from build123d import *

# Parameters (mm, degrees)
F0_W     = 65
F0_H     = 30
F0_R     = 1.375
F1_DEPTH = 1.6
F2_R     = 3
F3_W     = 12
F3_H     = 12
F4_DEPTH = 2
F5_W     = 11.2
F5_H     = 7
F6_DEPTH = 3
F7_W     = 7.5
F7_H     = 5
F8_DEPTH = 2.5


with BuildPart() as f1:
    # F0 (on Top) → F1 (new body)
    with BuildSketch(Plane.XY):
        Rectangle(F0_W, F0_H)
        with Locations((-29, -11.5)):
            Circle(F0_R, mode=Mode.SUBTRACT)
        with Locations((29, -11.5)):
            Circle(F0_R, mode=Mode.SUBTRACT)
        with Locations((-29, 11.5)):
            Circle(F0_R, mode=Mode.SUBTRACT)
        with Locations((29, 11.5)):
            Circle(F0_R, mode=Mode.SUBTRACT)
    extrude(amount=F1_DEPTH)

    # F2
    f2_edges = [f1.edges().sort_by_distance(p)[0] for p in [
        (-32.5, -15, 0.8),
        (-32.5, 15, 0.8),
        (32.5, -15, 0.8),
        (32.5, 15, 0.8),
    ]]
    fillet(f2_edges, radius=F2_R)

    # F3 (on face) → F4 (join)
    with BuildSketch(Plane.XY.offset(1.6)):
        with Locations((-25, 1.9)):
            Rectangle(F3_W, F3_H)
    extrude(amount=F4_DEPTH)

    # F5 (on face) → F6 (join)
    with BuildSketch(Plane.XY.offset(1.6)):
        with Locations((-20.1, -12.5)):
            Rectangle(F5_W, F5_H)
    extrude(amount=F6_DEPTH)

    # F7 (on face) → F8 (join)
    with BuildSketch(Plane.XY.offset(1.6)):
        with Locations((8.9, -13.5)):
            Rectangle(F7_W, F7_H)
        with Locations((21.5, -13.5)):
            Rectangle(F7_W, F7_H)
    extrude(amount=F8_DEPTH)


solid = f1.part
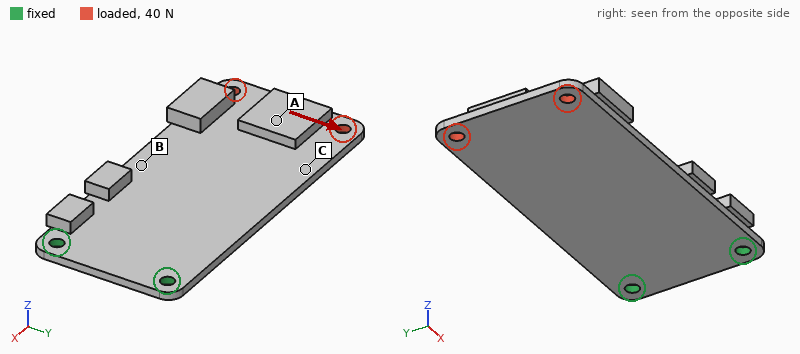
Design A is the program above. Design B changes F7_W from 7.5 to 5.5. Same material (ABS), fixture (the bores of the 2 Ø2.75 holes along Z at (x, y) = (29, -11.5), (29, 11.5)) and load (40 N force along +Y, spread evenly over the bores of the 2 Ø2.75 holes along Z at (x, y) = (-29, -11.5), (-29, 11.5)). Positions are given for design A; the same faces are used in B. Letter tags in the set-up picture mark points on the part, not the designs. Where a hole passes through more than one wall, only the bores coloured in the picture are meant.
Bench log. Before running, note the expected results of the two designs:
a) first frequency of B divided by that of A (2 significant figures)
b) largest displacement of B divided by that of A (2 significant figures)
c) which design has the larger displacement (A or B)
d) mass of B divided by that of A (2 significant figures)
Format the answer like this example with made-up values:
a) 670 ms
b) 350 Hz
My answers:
a) 0.97
b) 0.92
c) A
d) 0.99
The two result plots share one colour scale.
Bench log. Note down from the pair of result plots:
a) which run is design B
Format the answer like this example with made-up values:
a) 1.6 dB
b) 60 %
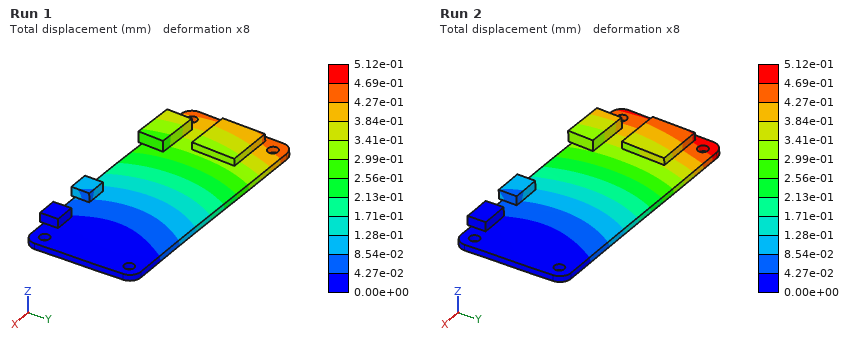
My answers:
a) Run 1
